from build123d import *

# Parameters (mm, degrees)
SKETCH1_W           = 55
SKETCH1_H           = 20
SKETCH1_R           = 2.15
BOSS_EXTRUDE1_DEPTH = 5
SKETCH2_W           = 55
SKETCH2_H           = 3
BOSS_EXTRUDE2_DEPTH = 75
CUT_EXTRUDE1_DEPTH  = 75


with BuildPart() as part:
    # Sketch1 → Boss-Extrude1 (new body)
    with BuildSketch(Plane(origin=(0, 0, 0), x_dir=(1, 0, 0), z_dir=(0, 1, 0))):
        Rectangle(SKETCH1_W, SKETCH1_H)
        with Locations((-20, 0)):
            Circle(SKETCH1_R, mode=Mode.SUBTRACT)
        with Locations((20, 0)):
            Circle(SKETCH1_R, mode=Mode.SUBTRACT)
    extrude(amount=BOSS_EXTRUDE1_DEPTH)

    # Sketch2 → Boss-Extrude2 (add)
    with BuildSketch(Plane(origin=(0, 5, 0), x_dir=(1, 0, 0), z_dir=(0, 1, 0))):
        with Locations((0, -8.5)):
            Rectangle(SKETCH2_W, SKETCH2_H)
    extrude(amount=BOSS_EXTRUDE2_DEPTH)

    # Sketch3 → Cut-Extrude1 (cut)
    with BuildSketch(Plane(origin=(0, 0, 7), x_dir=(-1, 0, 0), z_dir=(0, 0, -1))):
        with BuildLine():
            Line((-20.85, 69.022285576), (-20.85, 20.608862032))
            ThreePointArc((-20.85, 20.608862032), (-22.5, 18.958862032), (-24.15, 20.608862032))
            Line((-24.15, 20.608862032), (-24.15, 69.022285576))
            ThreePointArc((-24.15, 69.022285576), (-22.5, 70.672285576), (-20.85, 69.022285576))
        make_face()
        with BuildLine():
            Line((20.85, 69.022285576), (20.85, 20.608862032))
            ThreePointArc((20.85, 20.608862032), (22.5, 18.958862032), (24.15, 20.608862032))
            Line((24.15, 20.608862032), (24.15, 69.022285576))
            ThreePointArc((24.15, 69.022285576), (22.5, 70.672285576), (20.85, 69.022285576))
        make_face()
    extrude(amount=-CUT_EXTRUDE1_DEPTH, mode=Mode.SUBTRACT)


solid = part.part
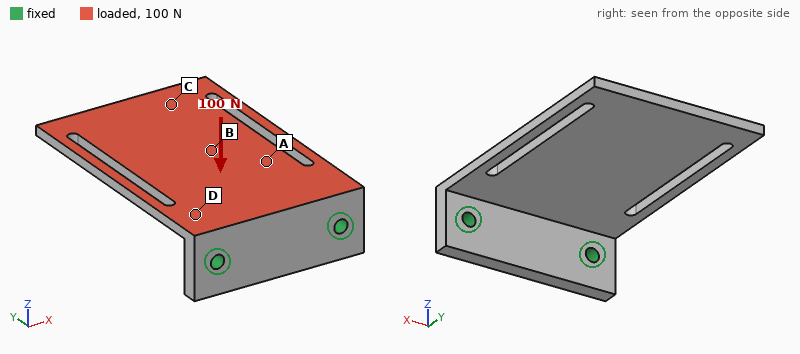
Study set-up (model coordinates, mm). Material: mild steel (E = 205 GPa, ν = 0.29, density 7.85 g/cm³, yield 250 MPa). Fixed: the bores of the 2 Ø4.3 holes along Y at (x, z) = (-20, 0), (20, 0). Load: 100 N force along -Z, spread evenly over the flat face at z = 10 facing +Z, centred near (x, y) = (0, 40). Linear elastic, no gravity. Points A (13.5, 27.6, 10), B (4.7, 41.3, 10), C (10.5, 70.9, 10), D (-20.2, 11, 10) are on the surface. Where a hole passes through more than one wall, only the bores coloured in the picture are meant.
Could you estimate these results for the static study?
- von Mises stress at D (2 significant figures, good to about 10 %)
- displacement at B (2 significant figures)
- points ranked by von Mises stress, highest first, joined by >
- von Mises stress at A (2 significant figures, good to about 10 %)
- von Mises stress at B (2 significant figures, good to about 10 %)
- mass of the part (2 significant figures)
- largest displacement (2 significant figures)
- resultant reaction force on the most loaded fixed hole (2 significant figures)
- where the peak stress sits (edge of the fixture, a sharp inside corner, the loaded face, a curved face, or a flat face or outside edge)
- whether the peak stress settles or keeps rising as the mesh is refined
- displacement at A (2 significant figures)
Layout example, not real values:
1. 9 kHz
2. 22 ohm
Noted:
1. 33 MPa
2. 0.084 mm
3. D > A > B > C
4. 22 MPa
5. 12 MPa
6. 130 g
7. 0.24 mm
8. 50 N
9. edge of the fixture
10. keeps rising
11. 0.040 mm
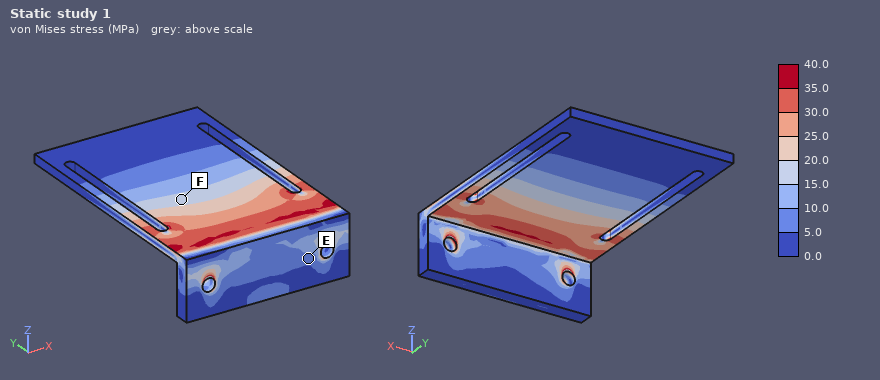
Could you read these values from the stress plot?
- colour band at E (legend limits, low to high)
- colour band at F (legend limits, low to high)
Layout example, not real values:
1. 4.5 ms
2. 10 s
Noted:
1. 5.0 to 10.0 MPa
2. 15.0 to 20.0 MPa
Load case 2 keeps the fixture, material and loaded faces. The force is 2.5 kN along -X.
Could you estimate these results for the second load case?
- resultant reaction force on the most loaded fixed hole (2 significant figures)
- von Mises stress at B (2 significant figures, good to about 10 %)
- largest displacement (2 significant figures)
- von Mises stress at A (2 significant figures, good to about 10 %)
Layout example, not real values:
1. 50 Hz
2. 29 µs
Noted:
1. 2.6 kN
2. 42 MPa
3. 94 µm
4. 45 MPa
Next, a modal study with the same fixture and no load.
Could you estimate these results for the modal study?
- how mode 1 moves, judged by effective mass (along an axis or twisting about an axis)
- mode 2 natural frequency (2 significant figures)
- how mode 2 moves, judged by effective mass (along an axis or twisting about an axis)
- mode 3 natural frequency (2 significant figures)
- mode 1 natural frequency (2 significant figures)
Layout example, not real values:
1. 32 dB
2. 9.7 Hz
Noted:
1. along Z
2. 1300 Hz
3. twisting about Y
4. 2500 Hz
5. 410 Hz
